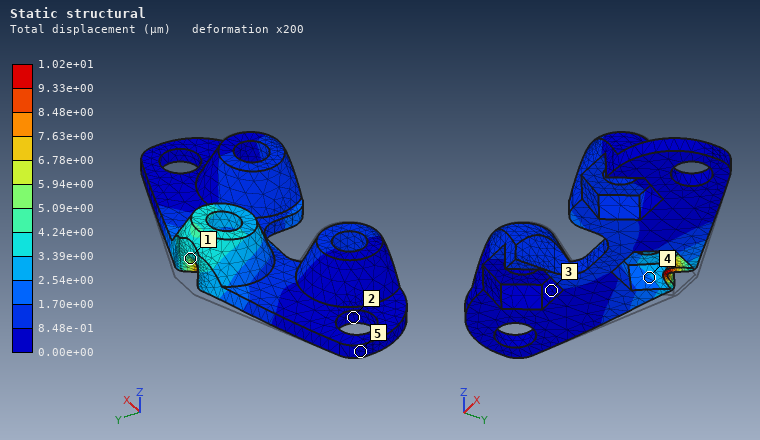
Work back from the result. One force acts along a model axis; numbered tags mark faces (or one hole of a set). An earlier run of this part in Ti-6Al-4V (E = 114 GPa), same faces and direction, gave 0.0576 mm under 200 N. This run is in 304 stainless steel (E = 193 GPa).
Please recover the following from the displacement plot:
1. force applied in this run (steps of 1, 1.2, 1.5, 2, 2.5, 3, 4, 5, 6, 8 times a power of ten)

60 N
